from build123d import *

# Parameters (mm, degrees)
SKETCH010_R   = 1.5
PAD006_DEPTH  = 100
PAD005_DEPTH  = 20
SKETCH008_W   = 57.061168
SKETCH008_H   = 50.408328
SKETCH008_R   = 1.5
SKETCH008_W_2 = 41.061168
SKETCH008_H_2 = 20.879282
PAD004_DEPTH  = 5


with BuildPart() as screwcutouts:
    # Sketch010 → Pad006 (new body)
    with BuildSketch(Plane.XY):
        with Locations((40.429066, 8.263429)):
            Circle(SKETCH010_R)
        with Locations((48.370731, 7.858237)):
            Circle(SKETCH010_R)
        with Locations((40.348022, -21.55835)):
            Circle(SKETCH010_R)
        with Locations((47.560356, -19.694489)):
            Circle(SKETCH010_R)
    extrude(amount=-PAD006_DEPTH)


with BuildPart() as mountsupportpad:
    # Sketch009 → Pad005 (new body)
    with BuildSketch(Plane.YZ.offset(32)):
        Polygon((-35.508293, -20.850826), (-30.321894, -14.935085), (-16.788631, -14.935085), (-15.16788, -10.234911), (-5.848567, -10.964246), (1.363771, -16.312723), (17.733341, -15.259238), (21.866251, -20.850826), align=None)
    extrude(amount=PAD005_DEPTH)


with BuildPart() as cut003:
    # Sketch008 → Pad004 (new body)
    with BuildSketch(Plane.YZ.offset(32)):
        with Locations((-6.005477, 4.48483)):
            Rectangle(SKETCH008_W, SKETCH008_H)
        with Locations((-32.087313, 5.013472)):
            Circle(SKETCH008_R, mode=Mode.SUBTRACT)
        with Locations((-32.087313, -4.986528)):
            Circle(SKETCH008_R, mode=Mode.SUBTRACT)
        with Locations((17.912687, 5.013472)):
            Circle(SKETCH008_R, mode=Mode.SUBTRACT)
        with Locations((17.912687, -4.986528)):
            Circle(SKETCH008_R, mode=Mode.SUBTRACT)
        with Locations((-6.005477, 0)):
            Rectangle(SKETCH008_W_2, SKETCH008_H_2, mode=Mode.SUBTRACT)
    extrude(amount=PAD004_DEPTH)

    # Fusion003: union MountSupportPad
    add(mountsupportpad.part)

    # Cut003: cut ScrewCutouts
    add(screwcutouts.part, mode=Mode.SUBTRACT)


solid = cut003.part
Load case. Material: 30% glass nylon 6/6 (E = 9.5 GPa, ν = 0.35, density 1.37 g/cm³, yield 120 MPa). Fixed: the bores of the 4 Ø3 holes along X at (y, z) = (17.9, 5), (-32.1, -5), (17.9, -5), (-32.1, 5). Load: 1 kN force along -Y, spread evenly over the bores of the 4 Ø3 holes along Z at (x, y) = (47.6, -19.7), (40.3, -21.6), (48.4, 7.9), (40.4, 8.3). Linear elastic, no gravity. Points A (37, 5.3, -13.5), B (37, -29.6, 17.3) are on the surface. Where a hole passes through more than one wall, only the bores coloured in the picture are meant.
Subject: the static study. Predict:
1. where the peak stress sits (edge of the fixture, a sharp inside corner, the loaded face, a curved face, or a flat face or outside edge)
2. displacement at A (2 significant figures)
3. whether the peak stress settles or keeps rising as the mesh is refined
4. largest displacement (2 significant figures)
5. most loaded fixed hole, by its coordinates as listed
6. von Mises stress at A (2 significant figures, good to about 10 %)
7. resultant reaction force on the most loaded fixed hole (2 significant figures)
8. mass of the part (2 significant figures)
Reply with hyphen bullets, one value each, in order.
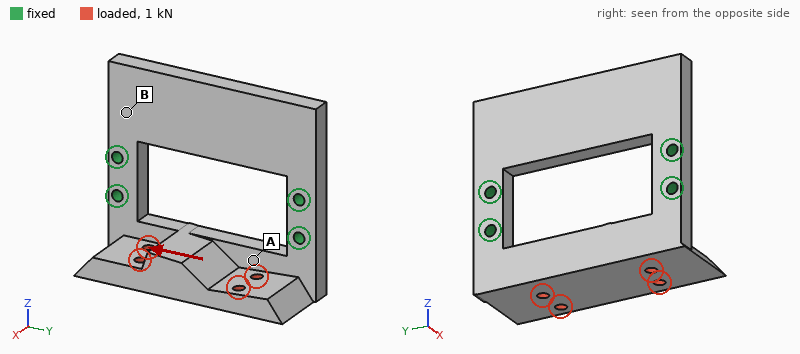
- edge of the fixture
- 0.081 mm
- keeps rising
- 0.18 mm
- (-32.1, -5)
- 19 MPa
- 690 N
- 21 g
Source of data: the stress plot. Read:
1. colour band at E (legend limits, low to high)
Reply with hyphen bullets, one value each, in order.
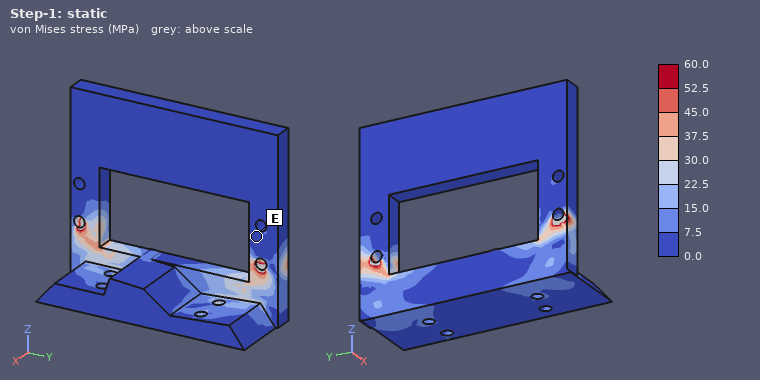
- 0.0 to 7.5 MPa
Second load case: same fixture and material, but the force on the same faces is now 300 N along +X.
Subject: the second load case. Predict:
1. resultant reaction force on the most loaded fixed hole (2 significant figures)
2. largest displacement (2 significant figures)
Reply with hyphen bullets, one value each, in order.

- 190 N
- 0.32 mm
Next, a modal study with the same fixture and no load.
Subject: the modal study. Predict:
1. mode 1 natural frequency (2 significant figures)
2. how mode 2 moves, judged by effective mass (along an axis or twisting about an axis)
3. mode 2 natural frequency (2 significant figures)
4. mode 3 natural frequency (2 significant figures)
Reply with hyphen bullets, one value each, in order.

- 1600 Hz
- along X
- 1800 Hz
- 4000 Hz
